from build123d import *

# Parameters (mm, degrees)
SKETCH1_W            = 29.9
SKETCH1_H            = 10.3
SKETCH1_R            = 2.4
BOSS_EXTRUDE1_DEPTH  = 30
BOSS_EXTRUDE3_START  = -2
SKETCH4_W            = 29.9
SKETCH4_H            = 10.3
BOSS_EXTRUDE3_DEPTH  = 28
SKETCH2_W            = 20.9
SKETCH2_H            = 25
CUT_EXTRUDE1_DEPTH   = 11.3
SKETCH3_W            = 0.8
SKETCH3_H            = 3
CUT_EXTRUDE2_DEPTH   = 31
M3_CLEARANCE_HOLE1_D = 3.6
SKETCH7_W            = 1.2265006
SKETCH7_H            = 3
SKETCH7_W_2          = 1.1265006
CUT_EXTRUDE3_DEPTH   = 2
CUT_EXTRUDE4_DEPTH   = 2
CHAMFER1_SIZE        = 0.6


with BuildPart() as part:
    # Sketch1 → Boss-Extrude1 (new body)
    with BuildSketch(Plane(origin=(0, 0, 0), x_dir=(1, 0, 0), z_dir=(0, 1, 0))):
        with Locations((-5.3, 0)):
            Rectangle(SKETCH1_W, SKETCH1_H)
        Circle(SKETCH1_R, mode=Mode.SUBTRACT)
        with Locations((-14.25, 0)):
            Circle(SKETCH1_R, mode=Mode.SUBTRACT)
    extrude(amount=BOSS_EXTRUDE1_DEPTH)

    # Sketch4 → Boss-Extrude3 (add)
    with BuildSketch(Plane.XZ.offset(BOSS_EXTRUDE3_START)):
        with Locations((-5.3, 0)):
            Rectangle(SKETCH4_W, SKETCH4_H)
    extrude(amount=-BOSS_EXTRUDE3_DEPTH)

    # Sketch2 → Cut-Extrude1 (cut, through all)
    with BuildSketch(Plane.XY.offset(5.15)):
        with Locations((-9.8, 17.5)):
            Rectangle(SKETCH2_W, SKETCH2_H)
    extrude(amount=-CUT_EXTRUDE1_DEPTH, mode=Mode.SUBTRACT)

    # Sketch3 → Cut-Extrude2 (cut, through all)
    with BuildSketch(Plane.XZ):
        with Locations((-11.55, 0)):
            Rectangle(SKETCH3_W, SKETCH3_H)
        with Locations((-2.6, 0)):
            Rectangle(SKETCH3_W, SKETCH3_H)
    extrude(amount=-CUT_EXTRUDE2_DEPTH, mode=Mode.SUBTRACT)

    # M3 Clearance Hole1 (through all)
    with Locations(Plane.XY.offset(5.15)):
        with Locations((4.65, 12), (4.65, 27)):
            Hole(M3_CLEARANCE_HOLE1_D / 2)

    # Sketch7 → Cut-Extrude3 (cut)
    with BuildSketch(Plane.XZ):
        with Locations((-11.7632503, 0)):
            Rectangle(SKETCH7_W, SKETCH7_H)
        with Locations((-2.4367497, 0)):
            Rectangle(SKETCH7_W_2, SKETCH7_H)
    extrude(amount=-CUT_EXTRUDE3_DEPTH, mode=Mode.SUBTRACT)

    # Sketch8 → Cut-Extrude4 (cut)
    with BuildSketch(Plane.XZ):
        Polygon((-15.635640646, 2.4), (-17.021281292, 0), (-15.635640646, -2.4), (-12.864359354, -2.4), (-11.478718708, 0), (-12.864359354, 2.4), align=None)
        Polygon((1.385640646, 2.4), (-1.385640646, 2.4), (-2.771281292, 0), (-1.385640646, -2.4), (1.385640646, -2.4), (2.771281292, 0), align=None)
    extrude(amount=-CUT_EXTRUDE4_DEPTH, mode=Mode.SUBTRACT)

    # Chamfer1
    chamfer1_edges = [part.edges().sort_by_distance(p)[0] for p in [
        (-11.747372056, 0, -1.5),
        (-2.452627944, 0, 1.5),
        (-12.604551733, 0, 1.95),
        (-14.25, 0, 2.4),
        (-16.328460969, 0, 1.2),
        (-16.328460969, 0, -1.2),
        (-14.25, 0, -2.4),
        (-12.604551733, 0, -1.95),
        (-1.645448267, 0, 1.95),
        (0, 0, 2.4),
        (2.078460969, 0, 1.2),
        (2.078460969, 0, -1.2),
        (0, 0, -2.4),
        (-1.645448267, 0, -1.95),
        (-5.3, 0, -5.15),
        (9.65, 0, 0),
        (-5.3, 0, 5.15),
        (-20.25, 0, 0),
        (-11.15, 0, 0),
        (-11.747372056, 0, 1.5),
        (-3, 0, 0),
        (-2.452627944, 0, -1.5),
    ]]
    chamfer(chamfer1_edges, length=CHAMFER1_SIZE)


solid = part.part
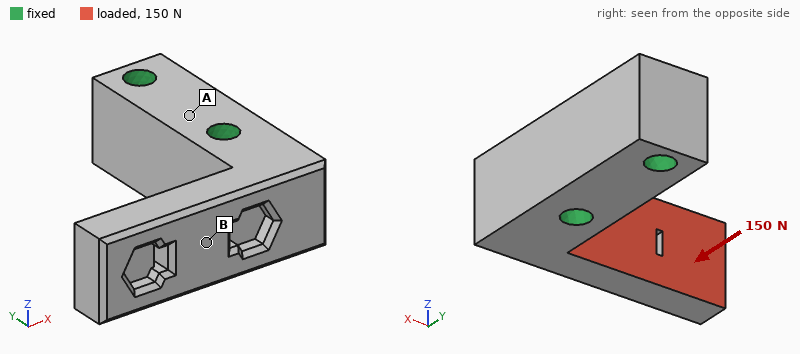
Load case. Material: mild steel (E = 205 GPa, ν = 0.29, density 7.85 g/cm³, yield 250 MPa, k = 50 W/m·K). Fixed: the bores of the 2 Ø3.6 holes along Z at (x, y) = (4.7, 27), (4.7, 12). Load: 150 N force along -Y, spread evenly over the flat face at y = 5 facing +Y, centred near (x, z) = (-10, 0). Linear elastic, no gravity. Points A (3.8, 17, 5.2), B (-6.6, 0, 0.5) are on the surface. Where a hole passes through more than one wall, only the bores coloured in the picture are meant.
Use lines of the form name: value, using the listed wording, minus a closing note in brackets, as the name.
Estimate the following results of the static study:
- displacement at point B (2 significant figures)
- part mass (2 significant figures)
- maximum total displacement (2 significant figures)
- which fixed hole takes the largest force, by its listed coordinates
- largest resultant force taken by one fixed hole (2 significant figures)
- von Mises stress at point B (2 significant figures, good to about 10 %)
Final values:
displacement at point B: 7.6 µm
part mass: 28 g
maximum total displacement: 22 µm
which fixed hole takes the largest force, by its listed coordinates: (4.7, 12)
largest resultant force taken by one fixed hole: 180 N
von Mises stress at point B: 12 MPa
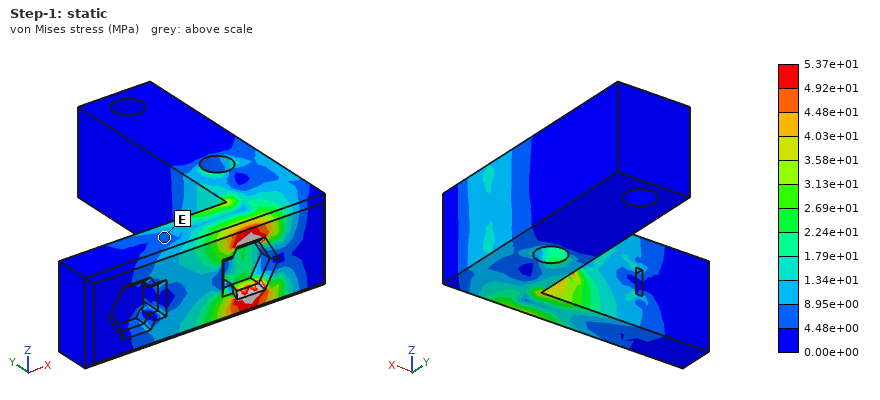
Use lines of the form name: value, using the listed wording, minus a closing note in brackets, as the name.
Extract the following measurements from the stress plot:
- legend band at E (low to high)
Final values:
legend band at E: 4.48e+00 to 8.95e+00 MPa
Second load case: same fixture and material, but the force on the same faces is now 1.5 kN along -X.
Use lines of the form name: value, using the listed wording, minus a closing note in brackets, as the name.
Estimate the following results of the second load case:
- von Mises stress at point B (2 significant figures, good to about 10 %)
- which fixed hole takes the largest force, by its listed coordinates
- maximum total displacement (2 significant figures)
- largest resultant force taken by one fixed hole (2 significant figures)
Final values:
von Mises stress at point B: 33 MPa
which fixed hole takes the largest force, by its listed coordinates: (4.7, 12)
maximum total displacement: 31 µm
largest resultant force taken by one fixed hole: 1.7 kN
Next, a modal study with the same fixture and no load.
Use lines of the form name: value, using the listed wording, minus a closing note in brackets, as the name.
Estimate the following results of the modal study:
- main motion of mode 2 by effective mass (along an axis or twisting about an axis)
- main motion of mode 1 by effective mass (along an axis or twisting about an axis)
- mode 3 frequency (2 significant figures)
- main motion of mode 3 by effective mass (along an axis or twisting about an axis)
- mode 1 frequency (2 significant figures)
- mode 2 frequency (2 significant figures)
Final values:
main motion of mode 2 by effective mass: along Z
main motion of mode 1 by effective mass: along Y
mode 3 frequency: 22 kHz
main motion of mode 3 by effective mass: along X
mode 1 frequency: 5900 Hz
mode 2 frequency: 9000 Hz
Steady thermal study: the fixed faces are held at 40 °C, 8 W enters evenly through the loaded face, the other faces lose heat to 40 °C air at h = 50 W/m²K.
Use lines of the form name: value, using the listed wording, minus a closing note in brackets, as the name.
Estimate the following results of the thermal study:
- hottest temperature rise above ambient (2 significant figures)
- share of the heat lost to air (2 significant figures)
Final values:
hottest temperature rise above ambient: 52 K
share of the heat lost to air: 16 %
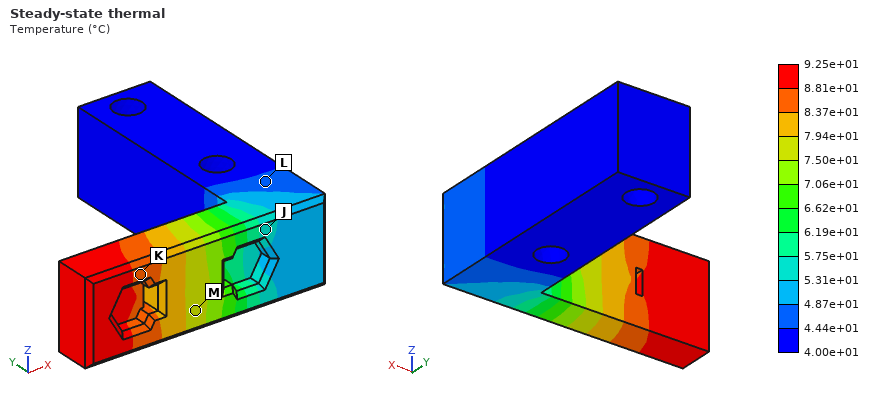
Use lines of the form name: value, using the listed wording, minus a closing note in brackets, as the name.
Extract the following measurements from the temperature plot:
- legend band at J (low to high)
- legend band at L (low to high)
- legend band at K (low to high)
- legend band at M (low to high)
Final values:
legend band at J: 5.31e+01 to 5.75e+01 °C
legend band at L: 4.44e+01 to 4.87e+01 °C
legend band at K: 8.37e+01 to 8.81e+01 °C
legend band at M: 7.50e+01 to 7.94e+01 °C
